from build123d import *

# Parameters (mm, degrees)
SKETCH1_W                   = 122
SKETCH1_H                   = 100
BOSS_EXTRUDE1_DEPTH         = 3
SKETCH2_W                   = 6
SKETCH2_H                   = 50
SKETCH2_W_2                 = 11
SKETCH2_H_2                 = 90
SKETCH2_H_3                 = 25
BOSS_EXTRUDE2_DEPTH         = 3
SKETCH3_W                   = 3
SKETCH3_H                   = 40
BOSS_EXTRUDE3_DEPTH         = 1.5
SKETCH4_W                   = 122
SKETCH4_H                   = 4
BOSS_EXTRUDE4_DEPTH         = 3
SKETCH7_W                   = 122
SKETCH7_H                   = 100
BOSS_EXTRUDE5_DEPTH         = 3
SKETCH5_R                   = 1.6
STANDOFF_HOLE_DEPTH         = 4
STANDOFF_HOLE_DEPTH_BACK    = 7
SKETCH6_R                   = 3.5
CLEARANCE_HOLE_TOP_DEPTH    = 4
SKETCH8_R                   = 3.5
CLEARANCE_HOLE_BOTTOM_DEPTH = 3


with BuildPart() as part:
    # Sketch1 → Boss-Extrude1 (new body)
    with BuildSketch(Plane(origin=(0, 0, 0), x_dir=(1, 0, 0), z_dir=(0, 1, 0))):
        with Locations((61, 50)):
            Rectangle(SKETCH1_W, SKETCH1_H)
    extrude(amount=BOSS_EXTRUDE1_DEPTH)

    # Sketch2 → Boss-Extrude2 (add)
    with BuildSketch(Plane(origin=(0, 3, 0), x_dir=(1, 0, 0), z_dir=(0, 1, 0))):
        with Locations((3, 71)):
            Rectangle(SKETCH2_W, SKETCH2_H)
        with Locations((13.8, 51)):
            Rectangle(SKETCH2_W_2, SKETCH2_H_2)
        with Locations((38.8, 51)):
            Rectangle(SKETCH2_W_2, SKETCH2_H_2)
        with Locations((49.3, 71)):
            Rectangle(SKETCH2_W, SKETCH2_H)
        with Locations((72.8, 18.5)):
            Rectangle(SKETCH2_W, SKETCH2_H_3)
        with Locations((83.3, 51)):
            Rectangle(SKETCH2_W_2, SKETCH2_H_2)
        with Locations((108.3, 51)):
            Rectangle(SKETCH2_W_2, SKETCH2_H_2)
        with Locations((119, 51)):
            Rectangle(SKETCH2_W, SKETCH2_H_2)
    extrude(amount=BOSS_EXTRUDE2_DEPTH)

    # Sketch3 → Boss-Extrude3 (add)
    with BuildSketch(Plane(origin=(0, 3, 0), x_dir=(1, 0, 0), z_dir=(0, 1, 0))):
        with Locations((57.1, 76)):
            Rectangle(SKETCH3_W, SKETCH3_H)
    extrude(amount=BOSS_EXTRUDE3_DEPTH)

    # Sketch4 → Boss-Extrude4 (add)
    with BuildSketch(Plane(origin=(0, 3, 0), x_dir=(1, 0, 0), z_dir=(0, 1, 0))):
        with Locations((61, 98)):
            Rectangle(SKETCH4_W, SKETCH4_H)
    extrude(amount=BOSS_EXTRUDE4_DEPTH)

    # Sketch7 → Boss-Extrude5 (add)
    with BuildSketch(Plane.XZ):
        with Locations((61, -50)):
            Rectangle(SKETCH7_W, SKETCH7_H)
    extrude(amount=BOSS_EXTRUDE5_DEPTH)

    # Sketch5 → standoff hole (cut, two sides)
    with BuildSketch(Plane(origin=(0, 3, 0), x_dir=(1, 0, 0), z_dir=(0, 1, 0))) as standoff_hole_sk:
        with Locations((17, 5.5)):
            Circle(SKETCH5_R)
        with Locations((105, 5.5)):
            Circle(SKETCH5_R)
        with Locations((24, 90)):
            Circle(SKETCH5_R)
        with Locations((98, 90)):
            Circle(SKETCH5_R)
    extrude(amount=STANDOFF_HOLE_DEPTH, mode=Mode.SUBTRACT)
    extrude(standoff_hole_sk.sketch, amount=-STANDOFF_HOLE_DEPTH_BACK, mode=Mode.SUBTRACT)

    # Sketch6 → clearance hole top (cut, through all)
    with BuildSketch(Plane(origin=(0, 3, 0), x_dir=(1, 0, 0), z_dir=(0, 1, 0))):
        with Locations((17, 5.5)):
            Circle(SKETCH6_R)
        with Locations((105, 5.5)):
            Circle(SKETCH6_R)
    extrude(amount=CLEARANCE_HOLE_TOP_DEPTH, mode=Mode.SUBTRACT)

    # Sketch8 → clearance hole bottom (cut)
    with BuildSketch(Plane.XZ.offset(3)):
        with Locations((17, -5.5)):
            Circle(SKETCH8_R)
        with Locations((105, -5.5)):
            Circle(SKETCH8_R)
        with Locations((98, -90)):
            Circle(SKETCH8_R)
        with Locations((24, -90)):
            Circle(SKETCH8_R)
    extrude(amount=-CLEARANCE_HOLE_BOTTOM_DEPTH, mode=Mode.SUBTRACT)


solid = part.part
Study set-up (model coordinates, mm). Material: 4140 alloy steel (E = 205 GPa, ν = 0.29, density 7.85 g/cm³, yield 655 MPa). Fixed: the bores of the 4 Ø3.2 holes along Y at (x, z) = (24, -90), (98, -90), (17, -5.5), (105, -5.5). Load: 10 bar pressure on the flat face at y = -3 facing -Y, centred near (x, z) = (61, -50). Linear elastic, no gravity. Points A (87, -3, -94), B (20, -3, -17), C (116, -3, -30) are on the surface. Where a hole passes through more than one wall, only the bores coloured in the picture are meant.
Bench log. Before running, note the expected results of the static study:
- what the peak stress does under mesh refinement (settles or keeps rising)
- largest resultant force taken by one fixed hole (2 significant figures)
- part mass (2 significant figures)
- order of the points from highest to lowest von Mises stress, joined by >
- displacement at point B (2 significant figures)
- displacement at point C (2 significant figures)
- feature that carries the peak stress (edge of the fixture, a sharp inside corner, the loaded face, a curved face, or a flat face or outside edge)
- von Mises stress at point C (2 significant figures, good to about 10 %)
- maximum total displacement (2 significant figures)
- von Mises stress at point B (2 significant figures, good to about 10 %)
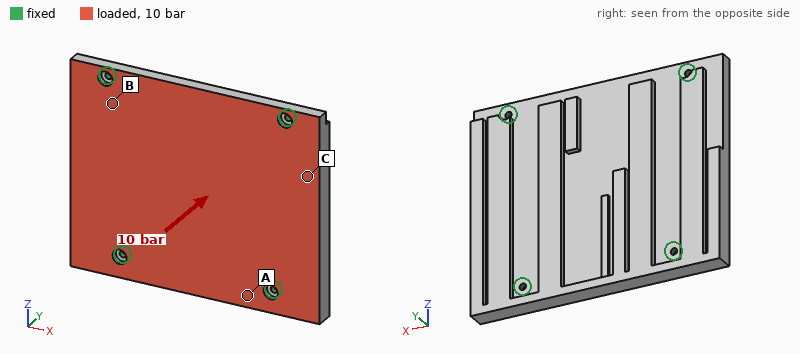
keeps rising
3.6 kN
710 g
B > C > A
0.034 mm
0.038 mm
edge of the fixture
51 MPa
0.11 mm
81 MPa
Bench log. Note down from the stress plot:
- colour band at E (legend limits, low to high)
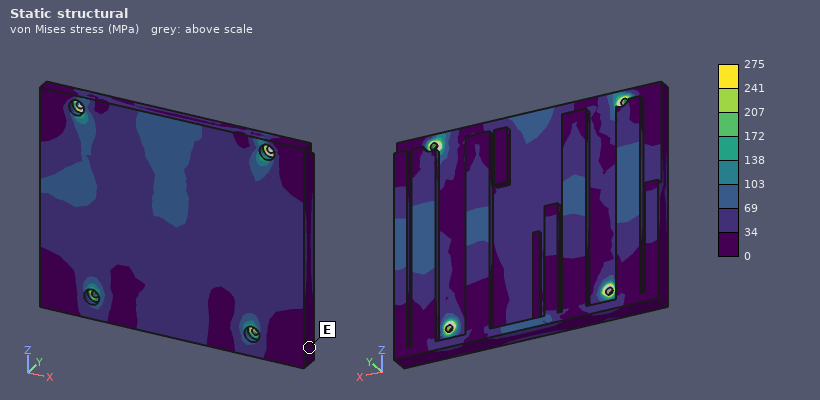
0 to 34 MPa
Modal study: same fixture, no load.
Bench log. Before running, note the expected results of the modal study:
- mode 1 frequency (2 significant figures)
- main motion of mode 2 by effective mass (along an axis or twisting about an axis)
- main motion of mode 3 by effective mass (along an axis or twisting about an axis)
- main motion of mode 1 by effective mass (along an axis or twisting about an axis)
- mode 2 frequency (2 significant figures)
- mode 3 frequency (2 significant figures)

2400 Hz
along Y
twisting about Z
along Y
3100 Hz
3300 Hz
